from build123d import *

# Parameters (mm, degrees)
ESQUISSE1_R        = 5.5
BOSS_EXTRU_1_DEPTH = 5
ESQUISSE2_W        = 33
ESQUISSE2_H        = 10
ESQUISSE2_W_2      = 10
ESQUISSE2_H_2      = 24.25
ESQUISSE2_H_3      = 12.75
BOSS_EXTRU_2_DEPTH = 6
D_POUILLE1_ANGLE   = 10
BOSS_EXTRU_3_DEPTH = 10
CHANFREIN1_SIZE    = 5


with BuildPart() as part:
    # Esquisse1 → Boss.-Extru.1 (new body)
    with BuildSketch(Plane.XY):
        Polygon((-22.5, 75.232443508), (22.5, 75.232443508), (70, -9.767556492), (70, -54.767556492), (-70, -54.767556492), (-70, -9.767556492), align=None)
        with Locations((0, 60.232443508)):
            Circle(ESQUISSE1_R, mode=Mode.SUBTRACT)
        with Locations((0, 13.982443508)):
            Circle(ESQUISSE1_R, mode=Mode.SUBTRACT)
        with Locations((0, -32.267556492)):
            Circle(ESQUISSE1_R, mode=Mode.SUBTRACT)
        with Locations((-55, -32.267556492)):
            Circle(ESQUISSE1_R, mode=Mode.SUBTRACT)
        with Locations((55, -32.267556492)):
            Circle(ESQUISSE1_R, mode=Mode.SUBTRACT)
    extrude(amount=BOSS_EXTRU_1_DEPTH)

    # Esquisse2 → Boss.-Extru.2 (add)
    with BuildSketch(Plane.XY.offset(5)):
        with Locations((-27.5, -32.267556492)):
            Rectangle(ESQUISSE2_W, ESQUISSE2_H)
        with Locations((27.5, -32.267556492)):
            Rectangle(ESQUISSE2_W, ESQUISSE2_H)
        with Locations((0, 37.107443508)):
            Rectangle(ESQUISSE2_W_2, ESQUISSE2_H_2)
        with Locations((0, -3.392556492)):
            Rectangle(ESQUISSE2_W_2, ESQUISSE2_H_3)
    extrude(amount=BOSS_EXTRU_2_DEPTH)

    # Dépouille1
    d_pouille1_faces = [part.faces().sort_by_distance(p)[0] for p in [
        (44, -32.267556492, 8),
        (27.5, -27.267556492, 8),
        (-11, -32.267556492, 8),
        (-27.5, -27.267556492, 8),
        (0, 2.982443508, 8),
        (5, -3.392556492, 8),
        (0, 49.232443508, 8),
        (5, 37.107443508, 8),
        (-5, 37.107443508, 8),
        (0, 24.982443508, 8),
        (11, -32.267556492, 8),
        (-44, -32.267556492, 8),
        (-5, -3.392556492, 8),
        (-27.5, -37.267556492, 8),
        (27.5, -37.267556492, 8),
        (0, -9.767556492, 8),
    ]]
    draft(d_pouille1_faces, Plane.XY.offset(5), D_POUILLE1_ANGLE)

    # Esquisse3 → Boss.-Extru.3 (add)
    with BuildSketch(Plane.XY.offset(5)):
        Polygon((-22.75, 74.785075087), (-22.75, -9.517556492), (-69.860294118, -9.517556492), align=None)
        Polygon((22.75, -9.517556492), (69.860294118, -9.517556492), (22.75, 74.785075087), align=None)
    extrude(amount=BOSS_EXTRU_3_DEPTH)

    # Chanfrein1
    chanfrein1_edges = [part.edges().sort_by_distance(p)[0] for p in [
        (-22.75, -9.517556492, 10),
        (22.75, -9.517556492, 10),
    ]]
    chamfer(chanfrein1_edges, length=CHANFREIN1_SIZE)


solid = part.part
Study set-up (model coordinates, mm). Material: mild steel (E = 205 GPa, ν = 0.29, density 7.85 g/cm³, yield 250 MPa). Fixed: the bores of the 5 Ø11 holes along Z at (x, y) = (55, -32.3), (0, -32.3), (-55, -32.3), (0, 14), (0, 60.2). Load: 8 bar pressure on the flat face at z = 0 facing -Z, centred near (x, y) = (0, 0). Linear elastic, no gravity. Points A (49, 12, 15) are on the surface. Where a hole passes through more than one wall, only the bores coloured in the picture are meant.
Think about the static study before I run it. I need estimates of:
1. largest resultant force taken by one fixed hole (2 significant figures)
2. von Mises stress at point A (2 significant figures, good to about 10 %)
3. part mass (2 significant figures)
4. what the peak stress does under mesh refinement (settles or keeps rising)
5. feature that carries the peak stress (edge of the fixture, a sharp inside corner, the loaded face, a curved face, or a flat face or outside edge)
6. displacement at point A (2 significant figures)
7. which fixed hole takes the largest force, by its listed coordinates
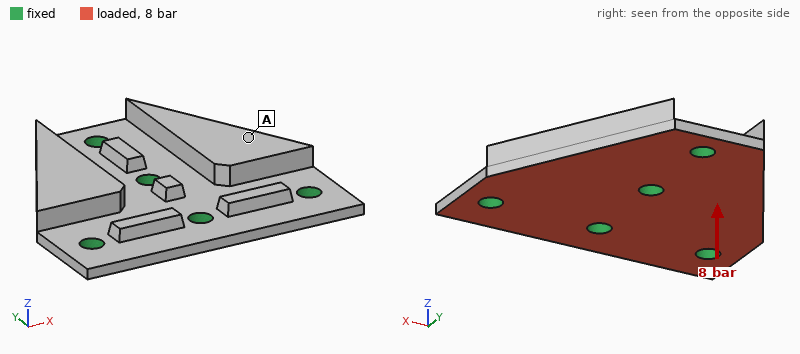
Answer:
2.8 kN
16 MPa
890 g
keeps rising
edge of the fixture
28 µm
(0, 60.2)
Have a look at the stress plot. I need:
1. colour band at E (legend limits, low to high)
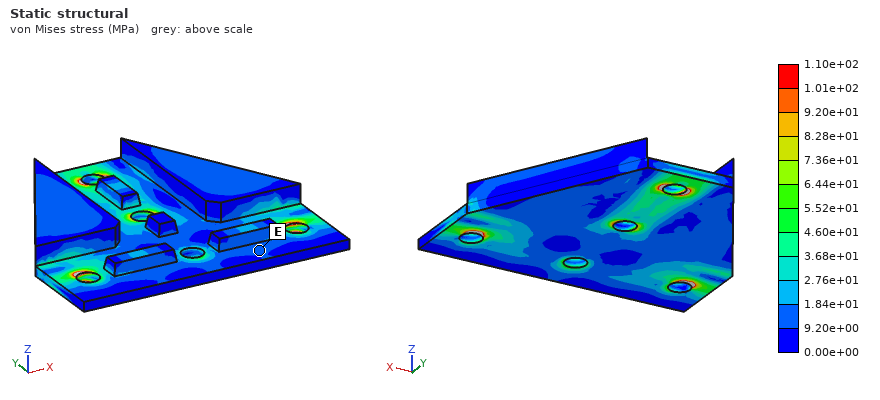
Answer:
9.20e+00 to 1.84e+01 MPa
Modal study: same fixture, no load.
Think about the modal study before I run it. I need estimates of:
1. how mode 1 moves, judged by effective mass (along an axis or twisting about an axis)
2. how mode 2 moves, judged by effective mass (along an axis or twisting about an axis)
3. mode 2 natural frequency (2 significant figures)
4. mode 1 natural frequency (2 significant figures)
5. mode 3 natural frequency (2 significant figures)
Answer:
twisting about Y
along Z
2900 Hz
2800 Hz
6400 Hz
